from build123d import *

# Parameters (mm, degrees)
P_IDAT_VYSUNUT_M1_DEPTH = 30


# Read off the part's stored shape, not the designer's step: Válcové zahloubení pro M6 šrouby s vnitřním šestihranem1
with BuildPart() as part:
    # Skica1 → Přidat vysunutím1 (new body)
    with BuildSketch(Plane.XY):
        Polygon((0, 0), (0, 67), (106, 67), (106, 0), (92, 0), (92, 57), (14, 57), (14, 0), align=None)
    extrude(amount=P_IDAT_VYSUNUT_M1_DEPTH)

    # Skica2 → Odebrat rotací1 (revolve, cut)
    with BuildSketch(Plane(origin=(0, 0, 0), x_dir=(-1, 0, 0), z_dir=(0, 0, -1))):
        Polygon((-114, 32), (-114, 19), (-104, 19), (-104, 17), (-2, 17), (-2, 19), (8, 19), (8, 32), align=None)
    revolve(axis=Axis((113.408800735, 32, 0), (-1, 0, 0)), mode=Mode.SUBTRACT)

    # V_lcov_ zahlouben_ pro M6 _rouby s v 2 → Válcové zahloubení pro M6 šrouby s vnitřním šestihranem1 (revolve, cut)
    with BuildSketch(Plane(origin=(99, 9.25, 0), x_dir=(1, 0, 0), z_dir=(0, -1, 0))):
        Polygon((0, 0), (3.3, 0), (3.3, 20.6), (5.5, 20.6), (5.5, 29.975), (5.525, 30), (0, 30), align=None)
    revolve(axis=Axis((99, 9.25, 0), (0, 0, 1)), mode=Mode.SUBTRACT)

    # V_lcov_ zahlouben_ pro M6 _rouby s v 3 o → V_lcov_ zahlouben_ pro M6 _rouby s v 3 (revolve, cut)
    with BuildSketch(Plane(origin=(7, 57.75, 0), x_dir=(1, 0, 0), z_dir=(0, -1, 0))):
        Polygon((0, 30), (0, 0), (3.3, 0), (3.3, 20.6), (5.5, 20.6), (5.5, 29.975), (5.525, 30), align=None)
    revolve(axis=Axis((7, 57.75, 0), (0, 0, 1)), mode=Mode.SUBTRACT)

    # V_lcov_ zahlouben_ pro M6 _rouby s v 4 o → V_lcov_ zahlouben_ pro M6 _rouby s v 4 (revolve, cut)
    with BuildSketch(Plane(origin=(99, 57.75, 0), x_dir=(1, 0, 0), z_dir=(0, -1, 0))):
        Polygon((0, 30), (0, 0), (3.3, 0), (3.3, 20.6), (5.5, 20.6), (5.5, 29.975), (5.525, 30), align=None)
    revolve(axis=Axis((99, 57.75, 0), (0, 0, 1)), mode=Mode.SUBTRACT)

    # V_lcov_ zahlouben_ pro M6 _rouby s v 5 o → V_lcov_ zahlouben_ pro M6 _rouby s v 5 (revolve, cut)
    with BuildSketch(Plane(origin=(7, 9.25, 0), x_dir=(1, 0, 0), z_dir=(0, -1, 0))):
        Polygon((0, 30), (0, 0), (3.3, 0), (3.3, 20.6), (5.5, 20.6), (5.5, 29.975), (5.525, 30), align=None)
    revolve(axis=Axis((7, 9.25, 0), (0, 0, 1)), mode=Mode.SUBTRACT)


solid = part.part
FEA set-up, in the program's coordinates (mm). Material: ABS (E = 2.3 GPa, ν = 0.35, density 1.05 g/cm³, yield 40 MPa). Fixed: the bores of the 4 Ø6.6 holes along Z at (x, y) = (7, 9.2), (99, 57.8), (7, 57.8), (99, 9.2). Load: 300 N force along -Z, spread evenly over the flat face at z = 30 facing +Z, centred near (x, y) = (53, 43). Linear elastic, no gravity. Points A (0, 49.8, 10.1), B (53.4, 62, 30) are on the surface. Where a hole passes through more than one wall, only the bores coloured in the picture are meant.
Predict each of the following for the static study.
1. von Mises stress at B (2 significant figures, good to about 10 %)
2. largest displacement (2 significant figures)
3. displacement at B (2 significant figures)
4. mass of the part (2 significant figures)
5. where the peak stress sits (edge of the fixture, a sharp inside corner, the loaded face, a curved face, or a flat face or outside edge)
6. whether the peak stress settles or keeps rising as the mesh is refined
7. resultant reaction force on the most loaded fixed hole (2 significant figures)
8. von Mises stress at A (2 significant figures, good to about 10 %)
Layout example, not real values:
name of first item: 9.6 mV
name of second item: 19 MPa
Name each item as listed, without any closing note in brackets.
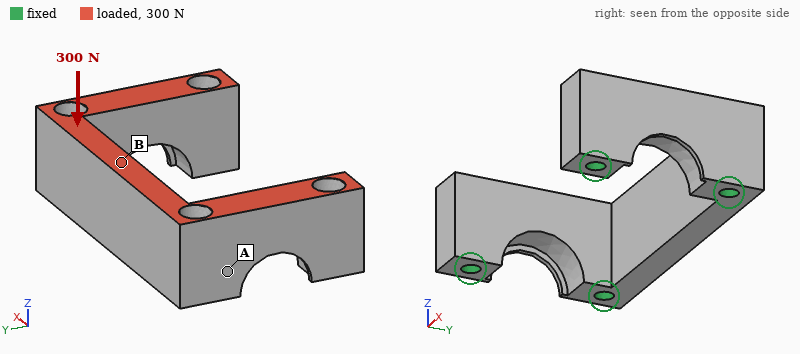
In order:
von Mises stress at B: 0.44 MPa
largest displacement: 13 µm
displacement at B: 13 µm
mass of the part: 67 g
where the peak stress sits: edge of the fixture
whether the peak stress settles or keeps rising as the mesh is refined: keeps rising
resultant reaction force on the most loaded fixed hole: 110 N
von Mises stress at A: 0.15 MPa
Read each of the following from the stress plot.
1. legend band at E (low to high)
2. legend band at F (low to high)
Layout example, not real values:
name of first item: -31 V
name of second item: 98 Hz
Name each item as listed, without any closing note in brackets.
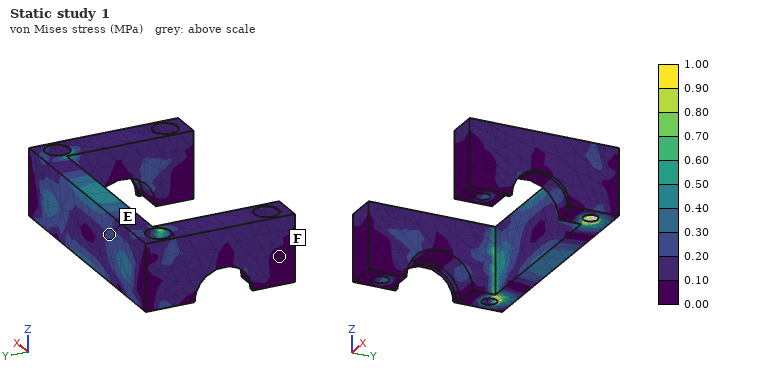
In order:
legend band at E: 0.20 to 0.30 MPa
legend band at F: 0.00 to 0.10 MPa
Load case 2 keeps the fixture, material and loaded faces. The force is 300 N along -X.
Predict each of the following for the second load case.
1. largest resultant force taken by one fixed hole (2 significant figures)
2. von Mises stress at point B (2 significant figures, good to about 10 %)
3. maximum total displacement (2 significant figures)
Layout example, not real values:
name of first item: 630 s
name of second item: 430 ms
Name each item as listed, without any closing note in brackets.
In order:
largest resultant force taken by one fixed hole: 110 N
von Mises stress at point B: 0.23 MPa
maximum total displacement: 21 µm
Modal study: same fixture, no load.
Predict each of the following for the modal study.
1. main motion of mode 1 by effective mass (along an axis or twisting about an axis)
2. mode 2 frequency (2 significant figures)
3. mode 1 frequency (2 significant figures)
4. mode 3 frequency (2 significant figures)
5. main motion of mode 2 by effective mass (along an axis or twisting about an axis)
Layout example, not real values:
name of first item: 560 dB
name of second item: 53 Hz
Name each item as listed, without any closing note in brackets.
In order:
main motion of mode 1 by effective mass: along Y
mode 2 frequency: 3100 Hz
mode 1 frequency: 1800 Hz
mode 3 frequency: 3300 Hz
main motion of mode 2 by effective mass: along Z
